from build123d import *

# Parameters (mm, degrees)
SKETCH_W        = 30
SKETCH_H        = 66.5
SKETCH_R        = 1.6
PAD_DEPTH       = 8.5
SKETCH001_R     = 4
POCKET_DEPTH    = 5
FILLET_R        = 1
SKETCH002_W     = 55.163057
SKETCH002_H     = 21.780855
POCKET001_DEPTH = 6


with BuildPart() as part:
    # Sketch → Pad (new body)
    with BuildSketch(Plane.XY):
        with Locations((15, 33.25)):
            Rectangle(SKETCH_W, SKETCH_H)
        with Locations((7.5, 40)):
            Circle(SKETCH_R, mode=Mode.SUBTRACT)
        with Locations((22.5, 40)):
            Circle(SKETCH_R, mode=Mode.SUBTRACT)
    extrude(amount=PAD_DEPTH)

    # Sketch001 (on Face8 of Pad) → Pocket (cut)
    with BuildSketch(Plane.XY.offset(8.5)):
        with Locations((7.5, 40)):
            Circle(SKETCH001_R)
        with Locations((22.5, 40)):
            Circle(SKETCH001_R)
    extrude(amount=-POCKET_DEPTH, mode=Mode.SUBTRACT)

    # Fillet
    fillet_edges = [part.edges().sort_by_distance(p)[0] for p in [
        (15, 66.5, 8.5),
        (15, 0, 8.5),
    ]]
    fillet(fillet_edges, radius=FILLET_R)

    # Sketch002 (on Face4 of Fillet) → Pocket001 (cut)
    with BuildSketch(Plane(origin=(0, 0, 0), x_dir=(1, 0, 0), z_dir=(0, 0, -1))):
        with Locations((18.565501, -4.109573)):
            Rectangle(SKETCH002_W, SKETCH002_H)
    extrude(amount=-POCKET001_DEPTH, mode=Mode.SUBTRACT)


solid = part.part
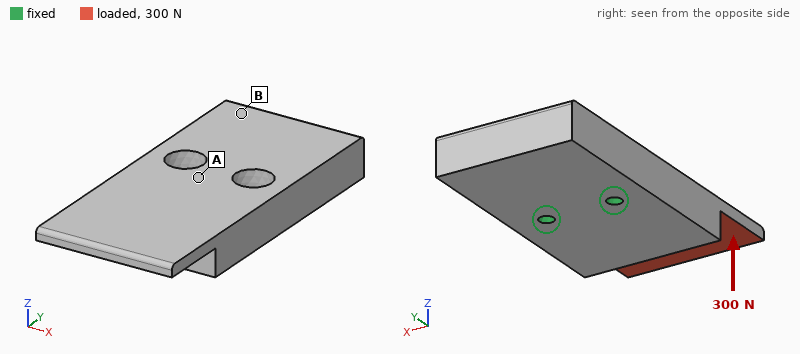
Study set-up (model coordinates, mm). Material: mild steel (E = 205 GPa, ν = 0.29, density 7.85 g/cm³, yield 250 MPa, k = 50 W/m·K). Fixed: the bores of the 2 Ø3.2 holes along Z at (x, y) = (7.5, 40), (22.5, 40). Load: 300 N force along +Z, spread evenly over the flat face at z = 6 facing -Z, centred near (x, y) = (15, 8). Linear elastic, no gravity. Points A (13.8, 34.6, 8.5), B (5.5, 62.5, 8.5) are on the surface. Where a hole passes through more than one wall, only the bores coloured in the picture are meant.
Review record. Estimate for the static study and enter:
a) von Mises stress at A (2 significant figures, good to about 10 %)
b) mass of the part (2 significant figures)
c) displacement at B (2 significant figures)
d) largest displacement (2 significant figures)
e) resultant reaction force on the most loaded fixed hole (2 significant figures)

31 MPa
110 g
16 µm
64 µm
160 N
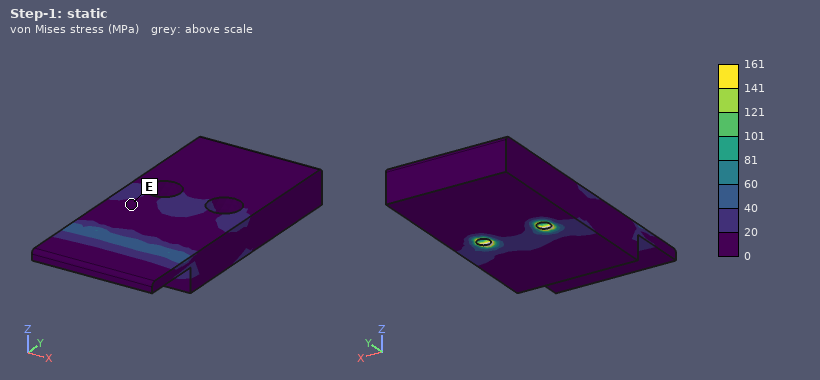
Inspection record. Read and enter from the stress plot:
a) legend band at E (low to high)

0 to 20 MPa
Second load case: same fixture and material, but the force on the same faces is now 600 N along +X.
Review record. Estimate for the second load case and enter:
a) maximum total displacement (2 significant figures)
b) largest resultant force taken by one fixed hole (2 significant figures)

11 µm
1.2 kN
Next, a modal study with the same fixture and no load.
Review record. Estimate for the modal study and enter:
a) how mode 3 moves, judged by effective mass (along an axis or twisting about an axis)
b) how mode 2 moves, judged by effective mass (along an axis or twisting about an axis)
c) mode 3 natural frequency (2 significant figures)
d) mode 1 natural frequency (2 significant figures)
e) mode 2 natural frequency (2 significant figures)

twisting about Z
along Z
9700 Hz
3000 Hz
6700 Hz
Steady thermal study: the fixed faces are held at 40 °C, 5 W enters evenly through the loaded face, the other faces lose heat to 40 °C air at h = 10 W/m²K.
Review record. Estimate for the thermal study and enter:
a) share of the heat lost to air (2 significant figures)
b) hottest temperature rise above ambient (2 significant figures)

6.4 %
23 K
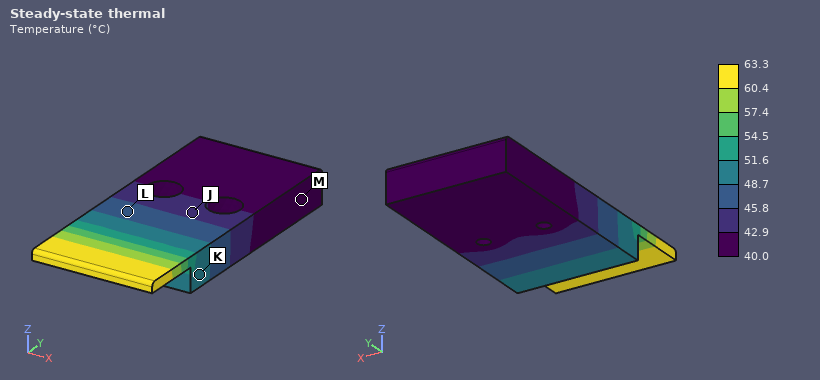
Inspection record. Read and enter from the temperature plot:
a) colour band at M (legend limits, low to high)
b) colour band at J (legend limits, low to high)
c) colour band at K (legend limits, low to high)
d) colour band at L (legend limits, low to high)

40.0 to 42.9 °C
42.9 to 45.8 °C
48.7 to 51.6 °C
45.8 to 48.7 °C
